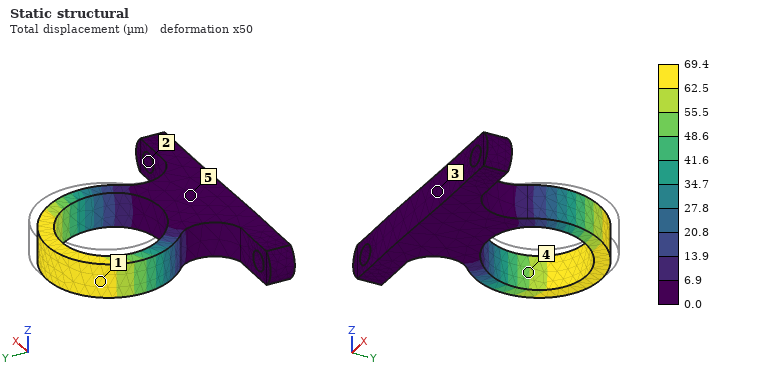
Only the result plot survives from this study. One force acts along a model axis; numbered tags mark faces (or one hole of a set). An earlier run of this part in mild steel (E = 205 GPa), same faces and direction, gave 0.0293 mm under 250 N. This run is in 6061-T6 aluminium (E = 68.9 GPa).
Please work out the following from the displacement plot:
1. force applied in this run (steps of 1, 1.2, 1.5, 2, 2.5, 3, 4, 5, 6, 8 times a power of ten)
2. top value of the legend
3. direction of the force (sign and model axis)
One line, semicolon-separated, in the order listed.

200 N; 69.4 µm; -X
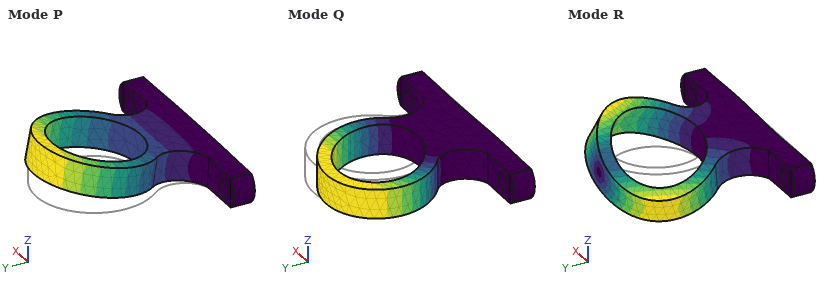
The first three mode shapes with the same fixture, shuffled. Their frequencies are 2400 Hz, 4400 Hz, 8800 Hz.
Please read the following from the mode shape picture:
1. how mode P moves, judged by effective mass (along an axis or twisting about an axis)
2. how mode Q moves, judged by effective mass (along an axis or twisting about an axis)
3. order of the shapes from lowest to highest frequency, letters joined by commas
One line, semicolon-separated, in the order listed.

along Z; along X; P, Q, R
